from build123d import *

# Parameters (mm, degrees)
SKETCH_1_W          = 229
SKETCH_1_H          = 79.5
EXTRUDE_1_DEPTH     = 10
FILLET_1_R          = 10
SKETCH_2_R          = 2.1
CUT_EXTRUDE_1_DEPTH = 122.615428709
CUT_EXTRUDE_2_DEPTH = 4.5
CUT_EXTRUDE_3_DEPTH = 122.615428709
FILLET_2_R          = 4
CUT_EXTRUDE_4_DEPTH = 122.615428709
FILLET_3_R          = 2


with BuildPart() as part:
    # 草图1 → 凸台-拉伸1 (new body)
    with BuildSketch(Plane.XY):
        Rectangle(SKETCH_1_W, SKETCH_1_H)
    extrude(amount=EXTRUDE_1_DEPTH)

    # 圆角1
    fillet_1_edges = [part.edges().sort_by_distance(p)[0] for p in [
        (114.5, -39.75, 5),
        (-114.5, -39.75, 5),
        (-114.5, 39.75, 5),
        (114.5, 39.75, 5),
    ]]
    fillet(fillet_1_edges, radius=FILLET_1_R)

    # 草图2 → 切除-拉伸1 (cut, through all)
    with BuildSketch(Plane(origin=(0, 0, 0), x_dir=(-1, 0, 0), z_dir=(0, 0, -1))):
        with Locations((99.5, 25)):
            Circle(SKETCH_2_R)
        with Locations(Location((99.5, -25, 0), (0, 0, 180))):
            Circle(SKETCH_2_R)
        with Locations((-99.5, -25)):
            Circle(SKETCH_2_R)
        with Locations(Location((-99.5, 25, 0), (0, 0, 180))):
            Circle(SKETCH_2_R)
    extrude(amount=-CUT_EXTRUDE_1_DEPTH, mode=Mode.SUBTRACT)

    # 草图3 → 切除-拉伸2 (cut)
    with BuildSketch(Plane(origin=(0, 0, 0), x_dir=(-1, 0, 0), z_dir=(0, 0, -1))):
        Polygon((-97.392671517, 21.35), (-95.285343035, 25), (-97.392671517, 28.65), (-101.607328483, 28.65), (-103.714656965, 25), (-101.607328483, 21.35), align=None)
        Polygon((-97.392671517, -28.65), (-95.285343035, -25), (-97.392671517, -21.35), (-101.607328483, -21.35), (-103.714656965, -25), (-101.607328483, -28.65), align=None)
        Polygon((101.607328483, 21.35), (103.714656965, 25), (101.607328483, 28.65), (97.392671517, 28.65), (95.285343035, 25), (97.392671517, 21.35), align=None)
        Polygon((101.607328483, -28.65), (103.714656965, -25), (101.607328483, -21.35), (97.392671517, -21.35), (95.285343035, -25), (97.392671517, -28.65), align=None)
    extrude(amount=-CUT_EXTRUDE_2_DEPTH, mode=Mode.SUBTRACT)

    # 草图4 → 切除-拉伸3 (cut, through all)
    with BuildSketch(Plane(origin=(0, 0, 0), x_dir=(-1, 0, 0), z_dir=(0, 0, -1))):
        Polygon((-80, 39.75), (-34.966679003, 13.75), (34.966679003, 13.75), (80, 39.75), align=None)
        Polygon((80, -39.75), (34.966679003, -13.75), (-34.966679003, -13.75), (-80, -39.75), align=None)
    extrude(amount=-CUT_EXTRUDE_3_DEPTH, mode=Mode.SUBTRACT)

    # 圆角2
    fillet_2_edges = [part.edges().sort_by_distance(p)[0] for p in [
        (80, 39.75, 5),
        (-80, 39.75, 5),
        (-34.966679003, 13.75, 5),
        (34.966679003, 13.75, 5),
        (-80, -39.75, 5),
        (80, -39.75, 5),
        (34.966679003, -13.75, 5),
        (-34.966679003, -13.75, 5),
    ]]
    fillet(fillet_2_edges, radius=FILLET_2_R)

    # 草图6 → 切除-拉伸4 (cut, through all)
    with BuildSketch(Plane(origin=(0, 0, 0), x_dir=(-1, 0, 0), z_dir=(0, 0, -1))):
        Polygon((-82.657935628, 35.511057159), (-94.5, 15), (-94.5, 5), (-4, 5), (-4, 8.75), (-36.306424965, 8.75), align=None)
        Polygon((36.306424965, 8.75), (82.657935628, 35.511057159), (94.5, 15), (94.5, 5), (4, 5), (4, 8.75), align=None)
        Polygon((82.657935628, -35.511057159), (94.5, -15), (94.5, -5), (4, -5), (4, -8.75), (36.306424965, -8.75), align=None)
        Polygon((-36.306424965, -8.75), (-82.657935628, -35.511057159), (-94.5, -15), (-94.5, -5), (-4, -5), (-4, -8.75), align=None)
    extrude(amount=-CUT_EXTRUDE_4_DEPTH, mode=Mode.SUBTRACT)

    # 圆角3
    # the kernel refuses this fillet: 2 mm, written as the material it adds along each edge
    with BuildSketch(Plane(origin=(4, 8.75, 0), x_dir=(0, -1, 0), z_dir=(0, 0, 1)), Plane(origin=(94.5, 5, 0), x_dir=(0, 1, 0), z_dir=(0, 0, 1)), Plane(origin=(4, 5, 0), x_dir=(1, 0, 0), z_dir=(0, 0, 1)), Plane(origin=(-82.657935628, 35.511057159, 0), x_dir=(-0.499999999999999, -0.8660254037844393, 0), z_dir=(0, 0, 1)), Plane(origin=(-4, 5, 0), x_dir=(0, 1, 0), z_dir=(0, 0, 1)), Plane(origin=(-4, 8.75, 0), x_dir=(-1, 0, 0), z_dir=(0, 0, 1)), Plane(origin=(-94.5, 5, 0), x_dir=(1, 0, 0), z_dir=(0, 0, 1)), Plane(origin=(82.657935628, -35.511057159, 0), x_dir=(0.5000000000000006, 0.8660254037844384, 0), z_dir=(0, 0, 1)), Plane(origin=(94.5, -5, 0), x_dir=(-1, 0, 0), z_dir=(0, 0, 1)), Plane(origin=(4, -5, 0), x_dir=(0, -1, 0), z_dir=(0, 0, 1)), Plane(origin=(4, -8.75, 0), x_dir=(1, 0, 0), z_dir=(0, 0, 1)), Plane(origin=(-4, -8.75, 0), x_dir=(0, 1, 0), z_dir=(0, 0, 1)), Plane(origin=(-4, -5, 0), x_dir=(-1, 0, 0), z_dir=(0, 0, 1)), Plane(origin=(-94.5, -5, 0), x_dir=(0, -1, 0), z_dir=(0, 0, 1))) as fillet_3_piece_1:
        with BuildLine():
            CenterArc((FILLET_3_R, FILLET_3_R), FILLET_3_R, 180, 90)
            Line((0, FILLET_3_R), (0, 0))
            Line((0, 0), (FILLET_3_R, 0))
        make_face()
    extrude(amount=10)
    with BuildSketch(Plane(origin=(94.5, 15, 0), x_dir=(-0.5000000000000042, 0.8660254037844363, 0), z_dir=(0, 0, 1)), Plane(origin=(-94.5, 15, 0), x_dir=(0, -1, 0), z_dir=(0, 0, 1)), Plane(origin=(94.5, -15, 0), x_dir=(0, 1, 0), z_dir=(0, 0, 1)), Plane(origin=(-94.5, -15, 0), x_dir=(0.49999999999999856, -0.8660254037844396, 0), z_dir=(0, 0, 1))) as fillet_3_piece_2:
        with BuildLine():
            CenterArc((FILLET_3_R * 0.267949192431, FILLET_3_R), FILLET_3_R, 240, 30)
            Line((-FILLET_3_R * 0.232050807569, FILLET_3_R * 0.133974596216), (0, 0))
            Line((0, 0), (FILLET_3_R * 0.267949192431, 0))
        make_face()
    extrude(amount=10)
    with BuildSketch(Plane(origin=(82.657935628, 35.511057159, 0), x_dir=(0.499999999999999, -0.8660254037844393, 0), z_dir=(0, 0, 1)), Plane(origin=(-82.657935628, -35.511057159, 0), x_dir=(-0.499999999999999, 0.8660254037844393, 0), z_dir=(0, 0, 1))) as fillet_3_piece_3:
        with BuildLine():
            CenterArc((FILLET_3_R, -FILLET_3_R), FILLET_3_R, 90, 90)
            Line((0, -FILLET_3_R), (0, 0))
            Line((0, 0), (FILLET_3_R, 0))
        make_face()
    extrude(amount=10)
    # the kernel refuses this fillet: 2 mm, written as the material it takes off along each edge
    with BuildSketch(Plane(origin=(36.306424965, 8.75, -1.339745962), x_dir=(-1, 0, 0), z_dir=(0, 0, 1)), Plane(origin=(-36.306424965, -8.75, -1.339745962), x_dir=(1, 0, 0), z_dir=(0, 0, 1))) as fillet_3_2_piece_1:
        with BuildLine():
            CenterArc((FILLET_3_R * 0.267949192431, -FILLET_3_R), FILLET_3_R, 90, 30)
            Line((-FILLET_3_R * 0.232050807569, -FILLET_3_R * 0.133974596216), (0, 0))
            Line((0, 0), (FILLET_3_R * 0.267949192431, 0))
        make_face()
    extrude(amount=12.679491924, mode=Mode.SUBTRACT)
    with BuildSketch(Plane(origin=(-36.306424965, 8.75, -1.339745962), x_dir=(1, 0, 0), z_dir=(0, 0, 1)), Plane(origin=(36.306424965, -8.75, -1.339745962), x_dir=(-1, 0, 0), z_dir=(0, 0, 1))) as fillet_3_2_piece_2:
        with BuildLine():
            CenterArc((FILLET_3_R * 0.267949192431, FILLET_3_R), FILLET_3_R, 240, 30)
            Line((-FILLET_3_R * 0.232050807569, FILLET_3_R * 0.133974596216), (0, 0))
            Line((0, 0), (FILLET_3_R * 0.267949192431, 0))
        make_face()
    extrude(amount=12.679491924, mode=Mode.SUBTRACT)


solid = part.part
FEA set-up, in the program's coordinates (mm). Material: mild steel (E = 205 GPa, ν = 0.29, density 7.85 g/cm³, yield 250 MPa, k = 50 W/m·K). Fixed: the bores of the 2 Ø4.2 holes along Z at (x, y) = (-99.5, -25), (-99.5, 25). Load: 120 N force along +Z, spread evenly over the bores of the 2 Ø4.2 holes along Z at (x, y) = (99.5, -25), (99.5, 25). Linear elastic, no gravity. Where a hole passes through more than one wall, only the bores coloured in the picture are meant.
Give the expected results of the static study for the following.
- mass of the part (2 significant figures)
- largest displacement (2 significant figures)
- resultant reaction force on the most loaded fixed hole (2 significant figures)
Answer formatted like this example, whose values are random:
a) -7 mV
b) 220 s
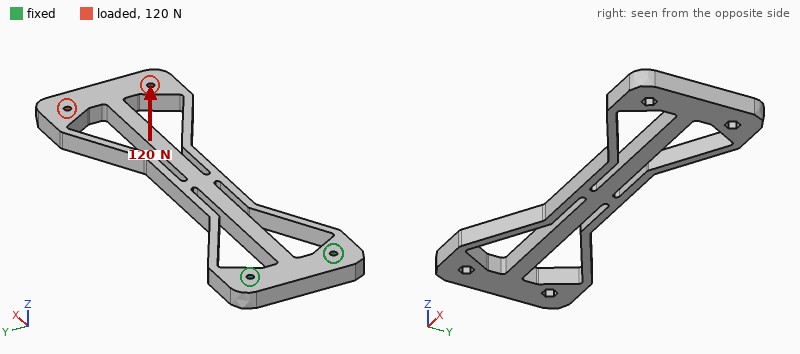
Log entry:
a) 580 g
b) 1.2 mm
c) 120 N
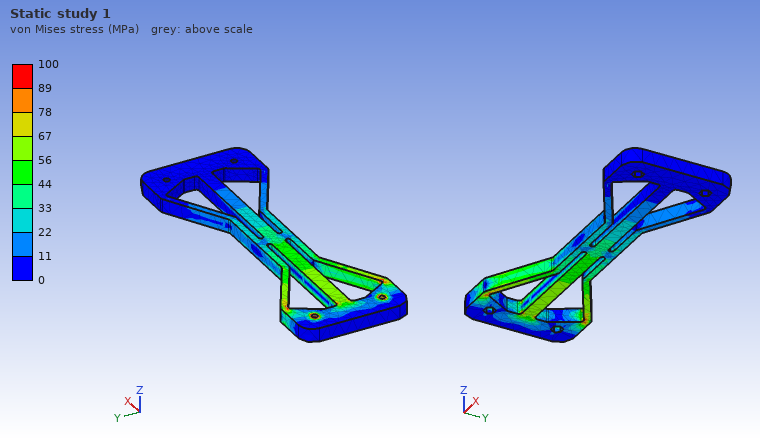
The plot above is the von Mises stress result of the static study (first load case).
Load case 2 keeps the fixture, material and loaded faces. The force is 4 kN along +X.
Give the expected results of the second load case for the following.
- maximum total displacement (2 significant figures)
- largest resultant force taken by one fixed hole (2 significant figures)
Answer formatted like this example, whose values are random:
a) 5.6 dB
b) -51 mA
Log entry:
a) 0.66 mm
b) 2.0 kN
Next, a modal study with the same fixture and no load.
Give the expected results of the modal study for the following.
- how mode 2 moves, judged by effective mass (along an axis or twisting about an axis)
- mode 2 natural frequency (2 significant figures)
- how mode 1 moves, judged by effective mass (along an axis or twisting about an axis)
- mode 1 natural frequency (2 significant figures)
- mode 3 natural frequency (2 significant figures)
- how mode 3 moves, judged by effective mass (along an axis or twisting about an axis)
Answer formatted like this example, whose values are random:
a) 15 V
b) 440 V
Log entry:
a) along Y
b) 220 Hz
c) along Z
d) 110 Hz
e) 500 Hz
f) twisting about X
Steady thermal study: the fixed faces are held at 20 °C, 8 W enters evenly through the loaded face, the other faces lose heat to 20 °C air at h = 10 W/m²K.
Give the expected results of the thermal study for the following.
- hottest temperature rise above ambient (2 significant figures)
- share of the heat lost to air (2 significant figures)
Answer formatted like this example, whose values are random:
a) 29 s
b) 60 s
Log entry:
a) 55 K
b) 83 %
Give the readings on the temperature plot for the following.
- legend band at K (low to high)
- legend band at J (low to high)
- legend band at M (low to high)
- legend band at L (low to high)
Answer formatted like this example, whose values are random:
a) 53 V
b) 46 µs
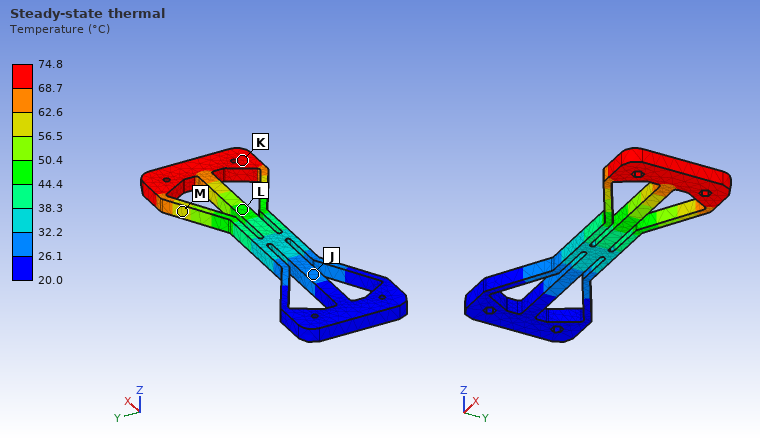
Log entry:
a) 68.7 to 74.8 °C
b) 26.1 to 32.2 °C
c) 56.5 to 62.6 °C
d) 44.4 to 50.4 °C
